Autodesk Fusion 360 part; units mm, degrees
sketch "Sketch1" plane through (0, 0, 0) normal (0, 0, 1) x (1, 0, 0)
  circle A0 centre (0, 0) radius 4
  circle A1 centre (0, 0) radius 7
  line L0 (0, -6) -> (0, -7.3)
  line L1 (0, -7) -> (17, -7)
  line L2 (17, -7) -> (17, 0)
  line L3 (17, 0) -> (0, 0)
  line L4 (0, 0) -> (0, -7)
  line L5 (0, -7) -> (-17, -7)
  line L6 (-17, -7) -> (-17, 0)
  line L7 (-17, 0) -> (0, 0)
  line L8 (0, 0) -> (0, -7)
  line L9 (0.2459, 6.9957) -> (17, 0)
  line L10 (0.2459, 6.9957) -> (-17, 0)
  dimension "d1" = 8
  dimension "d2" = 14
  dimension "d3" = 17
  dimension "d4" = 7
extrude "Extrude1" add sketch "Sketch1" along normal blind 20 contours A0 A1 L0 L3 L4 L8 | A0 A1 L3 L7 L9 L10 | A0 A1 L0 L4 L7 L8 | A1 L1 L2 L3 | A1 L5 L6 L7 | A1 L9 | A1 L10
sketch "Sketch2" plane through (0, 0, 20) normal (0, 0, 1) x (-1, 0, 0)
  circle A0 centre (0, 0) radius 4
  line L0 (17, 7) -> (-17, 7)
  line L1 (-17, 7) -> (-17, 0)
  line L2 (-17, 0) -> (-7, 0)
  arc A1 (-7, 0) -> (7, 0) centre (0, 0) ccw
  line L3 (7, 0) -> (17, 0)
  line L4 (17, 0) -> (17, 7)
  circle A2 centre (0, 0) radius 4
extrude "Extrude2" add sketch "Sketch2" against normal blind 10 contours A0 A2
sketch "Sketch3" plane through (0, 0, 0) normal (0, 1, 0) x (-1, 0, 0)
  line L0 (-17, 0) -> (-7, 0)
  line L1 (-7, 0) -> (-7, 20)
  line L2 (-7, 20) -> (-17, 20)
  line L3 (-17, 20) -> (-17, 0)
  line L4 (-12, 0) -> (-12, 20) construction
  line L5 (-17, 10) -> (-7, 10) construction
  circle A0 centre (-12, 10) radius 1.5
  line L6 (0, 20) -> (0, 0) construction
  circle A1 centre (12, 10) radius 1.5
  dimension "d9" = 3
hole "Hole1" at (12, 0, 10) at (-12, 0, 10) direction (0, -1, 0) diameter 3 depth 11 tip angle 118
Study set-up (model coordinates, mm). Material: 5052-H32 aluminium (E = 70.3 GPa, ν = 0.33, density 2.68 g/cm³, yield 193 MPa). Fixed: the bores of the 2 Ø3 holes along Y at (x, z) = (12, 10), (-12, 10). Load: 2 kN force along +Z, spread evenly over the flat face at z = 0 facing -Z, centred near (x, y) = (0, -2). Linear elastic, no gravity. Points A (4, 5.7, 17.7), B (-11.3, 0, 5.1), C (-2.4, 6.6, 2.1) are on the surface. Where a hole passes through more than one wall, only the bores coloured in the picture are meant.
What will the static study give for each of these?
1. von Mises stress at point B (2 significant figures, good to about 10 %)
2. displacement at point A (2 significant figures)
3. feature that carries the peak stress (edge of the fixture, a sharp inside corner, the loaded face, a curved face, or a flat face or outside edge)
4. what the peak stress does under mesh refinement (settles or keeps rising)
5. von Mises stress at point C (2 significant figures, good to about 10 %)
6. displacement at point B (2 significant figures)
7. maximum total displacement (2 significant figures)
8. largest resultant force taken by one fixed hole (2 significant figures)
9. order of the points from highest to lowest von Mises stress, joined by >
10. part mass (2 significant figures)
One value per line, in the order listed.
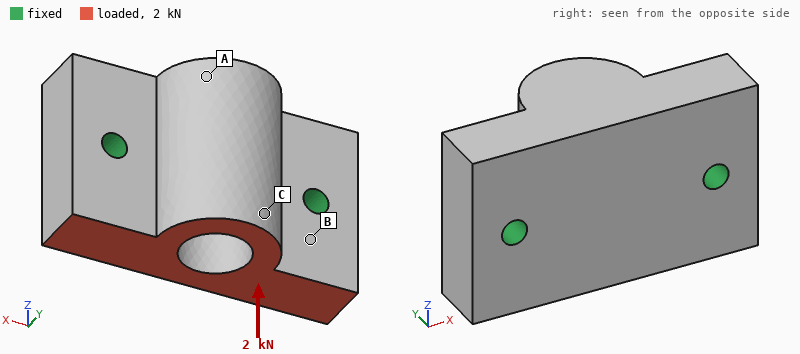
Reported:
16 MPa
4.6 µm
edge of the fixture
keeps rising
8.7 MPa
1.5 µm
6.6 µm
1.0 kN
B > C > A
15 g
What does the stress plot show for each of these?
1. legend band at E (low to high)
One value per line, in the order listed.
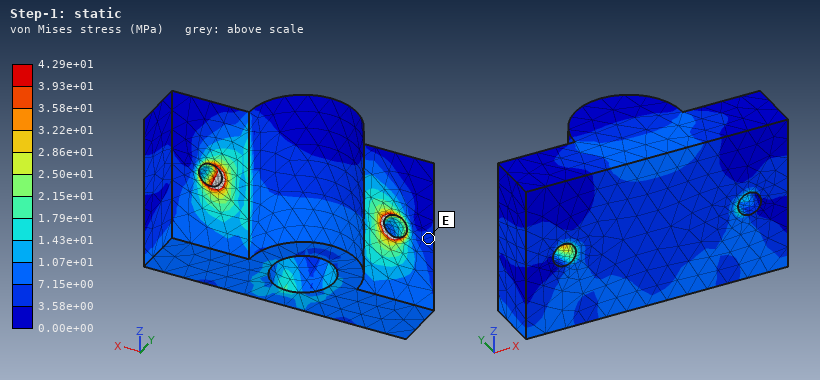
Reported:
3.58e+00 to 7.15e+00 MPa
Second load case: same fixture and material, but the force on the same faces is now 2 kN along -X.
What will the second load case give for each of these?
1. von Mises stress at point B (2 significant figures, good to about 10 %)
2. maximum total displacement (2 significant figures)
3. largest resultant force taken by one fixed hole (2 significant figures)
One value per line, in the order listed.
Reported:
19 MPa
8.3 µm
1.3 kN
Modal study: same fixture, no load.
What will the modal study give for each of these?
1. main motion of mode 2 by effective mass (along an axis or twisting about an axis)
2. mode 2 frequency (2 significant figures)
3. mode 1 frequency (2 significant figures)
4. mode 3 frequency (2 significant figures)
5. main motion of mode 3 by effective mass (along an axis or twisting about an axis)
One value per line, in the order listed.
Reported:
along Y
32 kHz
22 kHz
40 kHz
along Z
